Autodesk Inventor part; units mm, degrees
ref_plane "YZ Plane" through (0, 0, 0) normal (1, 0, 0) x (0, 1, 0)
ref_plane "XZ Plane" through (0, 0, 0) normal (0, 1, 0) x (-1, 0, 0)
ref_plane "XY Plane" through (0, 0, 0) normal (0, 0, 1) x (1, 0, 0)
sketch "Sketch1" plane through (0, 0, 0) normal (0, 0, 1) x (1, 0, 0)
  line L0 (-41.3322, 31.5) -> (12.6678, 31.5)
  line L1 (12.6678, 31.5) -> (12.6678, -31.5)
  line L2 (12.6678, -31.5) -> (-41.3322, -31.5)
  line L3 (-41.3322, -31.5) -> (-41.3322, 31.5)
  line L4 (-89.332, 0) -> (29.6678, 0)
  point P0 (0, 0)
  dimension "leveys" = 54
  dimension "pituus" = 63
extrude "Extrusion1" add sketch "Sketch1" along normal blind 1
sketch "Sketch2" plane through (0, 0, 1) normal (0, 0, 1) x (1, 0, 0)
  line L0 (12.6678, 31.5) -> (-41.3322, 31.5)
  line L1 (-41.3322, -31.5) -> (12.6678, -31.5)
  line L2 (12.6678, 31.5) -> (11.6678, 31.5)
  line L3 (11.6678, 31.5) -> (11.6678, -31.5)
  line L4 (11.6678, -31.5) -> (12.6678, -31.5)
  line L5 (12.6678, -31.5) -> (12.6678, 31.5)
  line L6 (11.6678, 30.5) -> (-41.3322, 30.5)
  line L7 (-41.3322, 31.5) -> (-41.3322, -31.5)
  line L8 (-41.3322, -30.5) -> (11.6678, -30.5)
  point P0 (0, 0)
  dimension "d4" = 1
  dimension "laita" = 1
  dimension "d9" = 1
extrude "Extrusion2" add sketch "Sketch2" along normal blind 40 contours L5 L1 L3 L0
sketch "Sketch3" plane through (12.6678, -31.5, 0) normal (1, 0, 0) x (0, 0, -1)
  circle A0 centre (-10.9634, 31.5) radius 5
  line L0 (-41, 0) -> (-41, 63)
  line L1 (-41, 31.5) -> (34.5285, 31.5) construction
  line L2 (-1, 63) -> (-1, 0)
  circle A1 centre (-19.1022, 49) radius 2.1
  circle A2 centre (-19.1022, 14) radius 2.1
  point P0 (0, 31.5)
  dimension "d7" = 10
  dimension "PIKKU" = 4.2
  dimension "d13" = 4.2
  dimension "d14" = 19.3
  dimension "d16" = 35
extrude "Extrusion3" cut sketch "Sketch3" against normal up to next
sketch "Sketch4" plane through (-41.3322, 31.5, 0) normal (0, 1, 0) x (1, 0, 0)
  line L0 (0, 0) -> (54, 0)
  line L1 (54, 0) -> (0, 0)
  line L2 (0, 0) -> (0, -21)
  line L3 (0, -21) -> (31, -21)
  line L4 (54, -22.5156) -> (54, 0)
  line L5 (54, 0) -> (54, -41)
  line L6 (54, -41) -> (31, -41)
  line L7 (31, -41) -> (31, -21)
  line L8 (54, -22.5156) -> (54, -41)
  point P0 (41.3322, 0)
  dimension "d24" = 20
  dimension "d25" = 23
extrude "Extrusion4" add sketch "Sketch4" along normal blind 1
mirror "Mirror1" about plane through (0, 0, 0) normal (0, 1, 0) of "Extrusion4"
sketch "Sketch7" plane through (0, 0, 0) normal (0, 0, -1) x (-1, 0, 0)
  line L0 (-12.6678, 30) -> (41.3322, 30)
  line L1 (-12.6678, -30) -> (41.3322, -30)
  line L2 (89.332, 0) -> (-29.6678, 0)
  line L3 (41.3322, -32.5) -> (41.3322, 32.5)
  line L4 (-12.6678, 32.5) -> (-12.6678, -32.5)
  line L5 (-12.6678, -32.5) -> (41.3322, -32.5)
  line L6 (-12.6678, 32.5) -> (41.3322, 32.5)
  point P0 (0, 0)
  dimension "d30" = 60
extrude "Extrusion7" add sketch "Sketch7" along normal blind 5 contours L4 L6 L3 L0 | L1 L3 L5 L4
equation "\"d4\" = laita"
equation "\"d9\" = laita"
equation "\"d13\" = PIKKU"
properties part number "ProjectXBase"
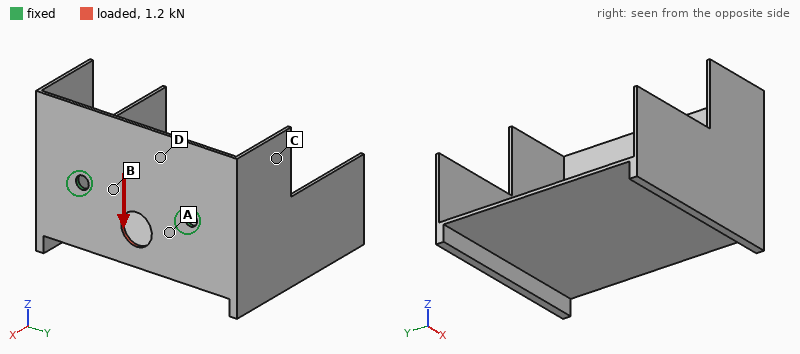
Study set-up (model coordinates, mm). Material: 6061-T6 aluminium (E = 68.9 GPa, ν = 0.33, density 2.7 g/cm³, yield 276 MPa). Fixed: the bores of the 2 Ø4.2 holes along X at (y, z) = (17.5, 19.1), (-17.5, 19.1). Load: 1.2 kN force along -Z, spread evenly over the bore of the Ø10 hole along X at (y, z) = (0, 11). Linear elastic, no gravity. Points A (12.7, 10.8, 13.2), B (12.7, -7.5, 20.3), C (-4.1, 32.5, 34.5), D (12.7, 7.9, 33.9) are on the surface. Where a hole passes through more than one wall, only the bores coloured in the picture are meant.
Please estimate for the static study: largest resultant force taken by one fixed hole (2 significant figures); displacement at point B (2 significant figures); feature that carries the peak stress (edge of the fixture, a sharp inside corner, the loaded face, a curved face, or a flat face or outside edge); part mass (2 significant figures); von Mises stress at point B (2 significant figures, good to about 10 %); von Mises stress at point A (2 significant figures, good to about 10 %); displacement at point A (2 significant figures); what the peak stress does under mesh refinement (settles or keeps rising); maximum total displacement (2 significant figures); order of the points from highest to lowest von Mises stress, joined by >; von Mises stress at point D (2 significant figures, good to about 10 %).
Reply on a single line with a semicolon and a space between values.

610 N; 8.7 µm; edge of the fixture; 28 g; 28 MPa; 42 MPa; 7.2 µm; keeps rising; 20 µm; A > B > D > C; 16 MPa
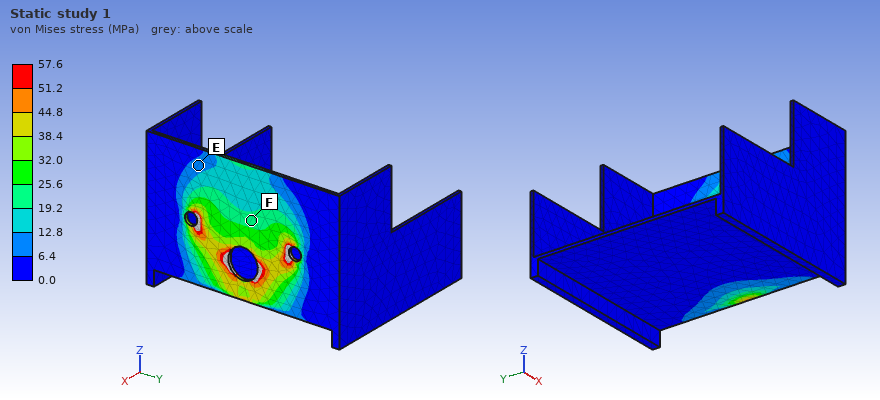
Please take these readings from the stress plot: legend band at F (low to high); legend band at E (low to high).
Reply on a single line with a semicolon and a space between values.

19.2 to 25.6 MPa; 6.4 to 12.8 MPa
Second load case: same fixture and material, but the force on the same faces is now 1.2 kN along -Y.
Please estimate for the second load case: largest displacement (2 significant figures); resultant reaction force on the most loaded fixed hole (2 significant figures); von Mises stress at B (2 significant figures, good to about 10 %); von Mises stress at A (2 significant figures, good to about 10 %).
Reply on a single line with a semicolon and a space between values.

19 µm; 650 N; 28 MPa; 48 MPa
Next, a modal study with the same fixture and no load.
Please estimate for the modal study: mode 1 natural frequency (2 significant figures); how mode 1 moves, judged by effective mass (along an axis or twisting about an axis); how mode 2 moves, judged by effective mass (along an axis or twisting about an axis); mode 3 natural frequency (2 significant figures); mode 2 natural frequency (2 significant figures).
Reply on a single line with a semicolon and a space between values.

280 Hz; along Z; along Y; 840 Hz; 360 Hz
